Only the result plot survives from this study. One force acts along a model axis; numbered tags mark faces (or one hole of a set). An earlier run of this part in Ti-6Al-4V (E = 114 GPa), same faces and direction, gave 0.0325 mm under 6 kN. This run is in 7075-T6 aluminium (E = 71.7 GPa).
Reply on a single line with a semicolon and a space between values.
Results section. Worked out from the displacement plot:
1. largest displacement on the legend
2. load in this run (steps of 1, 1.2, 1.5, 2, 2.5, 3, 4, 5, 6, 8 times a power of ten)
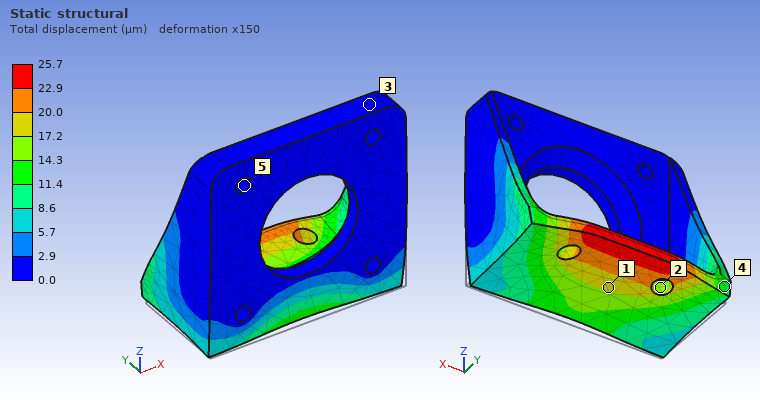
25.7 µm; 3 kN
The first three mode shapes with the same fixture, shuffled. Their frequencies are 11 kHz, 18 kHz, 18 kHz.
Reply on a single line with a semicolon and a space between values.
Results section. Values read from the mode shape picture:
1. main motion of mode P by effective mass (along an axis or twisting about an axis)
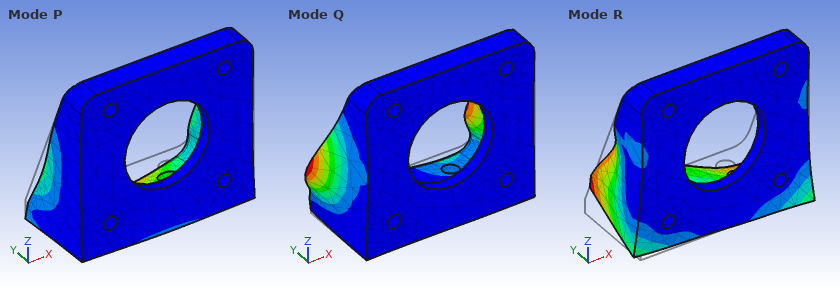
along Z
